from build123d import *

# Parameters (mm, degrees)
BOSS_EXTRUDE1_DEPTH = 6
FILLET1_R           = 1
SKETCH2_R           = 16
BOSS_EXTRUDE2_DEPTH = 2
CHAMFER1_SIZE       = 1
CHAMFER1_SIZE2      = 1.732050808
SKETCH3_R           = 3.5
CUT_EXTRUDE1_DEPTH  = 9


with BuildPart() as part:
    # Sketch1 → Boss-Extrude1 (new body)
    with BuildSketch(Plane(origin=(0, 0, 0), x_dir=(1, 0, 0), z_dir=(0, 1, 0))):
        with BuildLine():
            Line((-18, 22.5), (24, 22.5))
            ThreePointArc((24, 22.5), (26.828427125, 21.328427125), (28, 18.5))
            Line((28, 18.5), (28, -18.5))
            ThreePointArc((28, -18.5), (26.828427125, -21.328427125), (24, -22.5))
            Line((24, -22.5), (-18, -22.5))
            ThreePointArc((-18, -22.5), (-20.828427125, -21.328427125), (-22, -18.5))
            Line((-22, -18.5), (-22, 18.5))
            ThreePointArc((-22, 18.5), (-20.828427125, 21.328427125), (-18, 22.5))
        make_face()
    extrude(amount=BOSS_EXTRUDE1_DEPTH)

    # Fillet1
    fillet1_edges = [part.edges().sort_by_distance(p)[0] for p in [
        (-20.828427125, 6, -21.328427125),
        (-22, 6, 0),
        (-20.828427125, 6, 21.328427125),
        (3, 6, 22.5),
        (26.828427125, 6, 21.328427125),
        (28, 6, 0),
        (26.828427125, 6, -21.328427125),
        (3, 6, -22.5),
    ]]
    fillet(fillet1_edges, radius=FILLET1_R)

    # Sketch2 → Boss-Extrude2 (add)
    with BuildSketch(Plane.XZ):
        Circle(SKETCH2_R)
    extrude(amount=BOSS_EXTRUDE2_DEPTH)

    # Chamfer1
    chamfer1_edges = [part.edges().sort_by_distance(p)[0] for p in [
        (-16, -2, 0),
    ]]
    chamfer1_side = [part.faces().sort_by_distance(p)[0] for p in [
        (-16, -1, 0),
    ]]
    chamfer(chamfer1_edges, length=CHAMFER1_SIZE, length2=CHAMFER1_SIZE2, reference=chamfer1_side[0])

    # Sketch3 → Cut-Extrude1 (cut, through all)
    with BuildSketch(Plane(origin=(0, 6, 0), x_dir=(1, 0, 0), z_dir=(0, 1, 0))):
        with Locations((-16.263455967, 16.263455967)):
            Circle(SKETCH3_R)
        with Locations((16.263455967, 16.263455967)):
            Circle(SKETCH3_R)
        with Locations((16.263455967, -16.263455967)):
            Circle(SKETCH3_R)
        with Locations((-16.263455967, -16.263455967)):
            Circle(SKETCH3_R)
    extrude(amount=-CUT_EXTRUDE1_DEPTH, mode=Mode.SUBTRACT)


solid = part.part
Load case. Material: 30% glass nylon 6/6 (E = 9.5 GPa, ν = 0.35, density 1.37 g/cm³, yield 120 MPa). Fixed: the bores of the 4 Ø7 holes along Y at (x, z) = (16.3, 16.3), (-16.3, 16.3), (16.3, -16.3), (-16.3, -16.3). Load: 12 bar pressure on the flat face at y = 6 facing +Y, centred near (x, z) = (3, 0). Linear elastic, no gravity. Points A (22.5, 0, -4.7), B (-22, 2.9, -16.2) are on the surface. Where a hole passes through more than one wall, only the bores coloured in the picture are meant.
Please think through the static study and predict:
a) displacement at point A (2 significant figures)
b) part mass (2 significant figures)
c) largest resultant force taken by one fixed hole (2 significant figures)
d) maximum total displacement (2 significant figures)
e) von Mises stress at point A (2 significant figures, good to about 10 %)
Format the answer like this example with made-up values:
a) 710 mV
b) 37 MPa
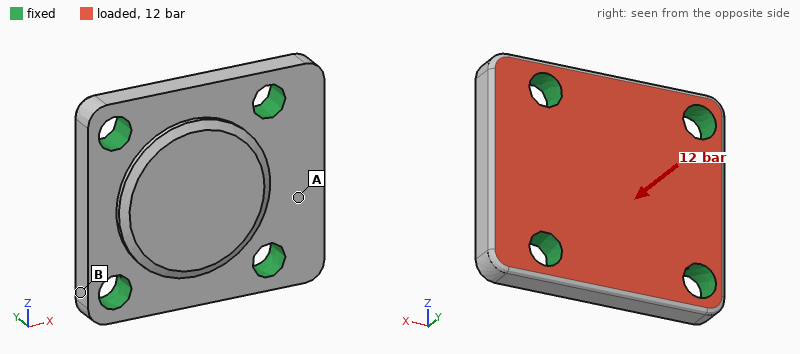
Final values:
a) 20 µm
b) 19 g
c) 660 N
d) 27 µm
e) 4.9 MPa
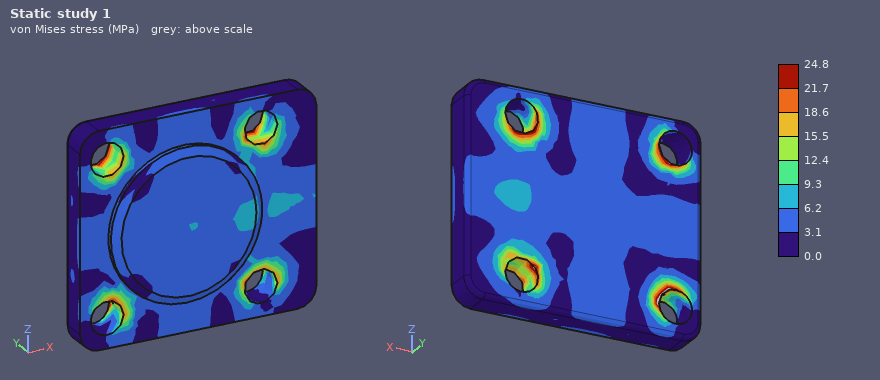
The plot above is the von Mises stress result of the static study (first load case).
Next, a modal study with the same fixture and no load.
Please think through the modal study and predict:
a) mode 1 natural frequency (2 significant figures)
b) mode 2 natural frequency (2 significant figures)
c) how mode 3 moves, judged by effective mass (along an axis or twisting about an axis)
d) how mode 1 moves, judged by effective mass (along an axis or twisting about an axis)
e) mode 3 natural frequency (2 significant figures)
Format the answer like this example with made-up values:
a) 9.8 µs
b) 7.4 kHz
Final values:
a) 12 kHz
b) 14 kHz
c) twisting about X
d) along Y
e) 18 kHz
